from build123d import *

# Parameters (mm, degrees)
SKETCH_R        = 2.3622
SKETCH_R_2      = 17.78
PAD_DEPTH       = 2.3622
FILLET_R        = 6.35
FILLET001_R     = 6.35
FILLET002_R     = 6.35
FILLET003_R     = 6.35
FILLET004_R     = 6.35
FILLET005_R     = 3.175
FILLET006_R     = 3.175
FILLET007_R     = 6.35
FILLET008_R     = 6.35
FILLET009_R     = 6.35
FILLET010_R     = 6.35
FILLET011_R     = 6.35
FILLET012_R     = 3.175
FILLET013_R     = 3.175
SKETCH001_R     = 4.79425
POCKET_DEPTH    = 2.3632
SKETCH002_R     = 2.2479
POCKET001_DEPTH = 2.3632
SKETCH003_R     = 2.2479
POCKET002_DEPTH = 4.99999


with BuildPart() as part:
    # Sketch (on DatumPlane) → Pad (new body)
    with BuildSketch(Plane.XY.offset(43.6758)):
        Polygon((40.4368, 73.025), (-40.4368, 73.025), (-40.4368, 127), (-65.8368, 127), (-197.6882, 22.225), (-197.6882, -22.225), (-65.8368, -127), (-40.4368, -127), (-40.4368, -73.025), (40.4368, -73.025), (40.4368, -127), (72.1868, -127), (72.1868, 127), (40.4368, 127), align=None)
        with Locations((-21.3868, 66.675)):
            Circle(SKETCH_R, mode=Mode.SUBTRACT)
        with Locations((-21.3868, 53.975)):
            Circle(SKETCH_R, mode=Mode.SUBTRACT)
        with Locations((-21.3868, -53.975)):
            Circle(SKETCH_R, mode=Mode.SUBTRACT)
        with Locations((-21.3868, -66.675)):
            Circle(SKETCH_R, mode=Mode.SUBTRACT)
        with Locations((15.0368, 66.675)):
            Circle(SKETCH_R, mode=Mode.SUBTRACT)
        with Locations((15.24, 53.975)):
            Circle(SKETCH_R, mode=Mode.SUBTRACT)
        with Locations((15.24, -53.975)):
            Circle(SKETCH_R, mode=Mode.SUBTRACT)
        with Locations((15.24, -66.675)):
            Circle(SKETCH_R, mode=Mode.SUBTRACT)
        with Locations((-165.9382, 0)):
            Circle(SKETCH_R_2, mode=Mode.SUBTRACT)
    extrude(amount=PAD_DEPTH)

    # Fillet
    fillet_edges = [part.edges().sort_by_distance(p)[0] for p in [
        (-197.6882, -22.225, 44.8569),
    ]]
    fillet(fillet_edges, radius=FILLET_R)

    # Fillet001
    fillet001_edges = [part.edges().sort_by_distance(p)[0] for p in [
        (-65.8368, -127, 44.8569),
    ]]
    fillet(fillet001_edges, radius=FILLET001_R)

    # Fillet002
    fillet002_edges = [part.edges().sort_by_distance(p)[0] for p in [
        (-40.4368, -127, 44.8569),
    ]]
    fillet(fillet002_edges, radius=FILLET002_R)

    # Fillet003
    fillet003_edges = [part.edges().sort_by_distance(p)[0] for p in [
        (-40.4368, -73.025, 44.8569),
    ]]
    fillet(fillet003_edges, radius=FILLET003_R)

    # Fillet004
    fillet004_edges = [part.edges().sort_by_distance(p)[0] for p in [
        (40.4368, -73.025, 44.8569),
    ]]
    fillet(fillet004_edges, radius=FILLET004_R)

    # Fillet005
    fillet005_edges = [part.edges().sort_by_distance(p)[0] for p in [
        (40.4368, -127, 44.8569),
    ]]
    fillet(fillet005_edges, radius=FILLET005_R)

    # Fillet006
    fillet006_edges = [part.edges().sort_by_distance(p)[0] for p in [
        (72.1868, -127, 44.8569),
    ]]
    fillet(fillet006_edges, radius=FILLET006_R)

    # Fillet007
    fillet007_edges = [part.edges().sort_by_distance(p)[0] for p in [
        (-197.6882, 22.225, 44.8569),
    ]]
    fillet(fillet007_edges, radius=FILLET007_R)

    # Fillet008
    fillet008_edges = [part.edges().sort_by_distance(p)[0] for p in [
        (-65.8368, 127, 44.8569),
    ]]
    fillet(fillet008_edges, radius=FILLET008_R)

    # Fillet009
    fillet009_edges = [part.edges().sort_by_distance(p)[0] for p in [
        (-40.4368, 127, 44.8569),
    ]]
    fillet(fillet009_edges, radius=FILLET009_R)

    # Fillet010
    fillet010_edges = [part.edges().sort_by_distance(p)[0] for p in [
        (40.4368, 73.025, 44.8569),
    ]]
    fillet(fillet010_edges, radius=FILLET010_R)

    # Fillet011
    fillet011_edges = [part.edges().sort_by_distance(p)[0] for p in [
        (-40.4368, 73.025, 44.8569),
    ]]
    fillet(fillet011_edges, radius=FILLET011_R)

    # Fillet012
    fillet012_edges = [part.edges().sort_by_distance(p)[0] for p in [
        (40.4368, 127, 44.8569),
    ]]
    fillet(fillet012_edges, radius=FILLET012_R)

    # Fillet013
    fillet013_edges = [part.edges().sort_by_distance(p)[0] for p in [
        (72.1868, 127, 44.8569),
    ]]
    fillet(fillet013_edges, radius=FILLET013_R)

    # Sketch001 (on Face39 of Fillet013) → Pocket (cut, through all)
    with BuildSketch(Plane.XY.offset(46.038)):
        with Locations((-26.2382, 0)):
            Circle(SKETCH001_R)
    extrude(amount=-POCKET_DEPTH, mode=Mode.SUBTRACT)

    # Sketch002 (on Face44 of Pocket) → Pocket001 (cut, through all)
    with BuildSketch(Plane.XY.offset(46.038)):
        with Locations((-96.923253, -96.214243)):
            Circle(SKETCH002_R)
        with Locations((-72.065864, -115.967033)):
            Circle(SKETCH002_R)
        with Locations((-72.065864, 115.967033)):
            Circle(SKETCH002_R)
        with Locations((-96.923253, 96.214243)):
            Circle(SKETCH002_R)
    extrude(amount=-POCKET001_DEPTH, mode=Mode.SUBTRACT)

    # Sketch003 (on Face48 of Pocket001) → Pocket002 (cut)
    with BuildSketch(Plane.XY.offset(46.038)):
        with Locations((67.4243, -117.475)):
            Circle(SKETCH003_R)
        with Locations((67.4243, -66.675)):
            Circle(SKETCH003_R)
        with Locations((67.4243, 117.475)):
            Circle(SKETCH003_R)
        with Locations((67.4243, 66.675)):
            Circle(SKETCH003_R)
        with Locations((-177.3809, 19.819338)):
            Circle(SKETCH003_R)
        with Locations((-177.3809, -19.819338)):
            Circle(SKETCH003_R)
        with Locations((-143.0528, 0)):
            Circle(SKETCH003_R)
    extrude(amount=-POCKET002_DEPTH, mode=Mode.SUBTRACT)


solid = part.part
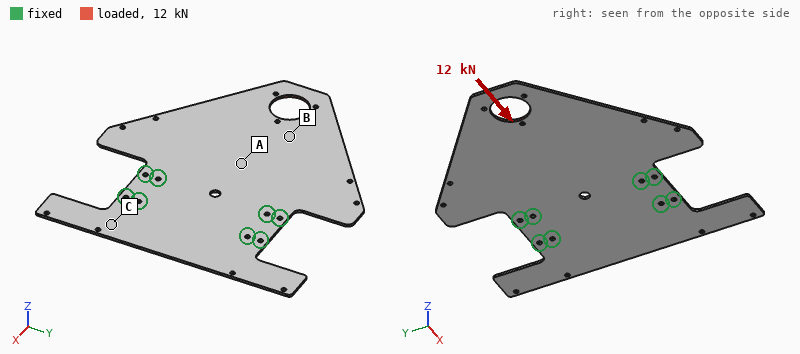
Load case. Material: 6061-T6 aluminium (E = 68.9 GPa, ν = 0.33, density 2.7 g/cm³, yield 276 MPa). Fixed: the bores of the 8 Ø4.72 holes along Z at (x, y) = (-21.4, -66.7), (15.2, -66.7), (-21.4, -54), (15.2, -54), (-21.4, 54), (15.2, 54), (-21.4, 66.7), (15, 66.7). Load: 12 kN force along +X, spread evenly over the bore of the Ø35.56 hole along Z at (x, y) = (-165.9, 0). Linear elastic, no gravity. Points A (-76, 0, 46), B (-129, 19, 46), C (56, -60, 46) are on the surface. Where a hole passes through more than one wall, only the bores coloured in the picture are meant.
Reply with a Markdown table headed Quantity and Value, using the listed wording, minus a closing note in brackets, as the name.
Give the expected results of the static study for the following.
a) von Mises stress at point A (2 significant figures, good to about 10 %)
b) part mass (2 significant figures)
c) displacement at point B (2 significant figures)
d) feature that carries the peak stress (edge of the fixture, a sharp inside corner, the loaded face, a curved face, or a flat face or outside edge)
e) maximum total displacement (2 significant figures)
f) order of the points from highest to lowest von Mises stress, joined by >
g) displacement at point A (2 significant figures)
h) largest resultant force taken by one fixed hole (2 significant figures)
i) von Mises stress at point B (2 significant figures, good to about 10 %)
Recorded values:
| Quantity | Value |
|---|---|
| von Mises stress at point A | 33 MPa |
| part mass | 280 g |
| displacement at point B | 0.071 mm |
| feature that carries the peak stress | a curved face |
| maximum total displacement | 0.16 mm |
| order of the points from highest to lowest von Mises stress, joined by > | B > A > C |
| displacement at point A | 0.040 mm |
| largest resultant force taken by one fixed hole | 2.6 kN |
| von Mises stress at point B | 52 MPa |
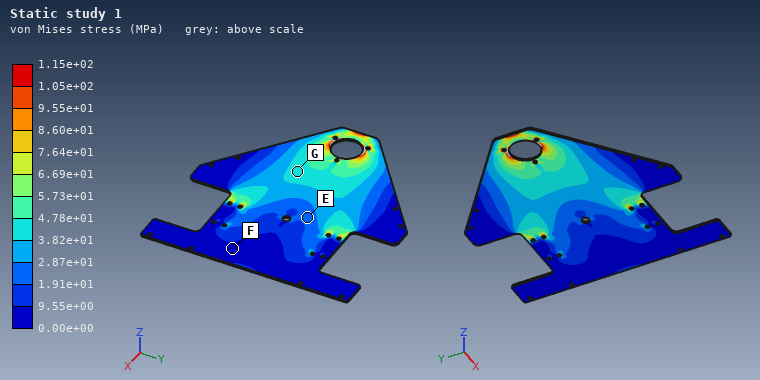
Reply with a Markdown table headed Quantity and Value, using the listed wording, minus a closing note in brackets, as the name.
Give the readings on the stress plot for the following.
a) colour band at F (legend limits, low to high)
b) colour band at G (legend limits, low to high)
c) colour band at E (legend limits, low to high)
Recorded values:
| Quantity | Value |
|---|---|
| colour band at F | 0.00e+00 to 9.55e+00 MPa |
| colour band at G | 3.82e+01 to 4.78e+01 MPa |
| colour band at E | 1.91e+01 to 2.87e+01 MPa |
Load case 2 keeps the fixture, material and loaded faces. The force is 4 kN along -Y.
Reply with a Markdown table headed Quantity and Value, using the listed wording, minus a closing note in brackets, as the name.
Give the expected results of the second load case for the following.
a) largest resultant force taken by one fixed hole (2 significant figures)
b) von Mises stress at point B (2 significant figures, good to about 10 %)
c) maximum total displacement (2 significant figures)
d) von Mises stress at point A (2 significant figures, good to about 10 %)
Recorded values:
| Quantity | Value |
|---|---|
| largest resultant force taken by one fixed hole | 2.6 kN |
| von Mises stress at point B | 22 MPa |
| maximum total displacement | 0.21 mm |
| von Mises stress at point A | 29 MPa |
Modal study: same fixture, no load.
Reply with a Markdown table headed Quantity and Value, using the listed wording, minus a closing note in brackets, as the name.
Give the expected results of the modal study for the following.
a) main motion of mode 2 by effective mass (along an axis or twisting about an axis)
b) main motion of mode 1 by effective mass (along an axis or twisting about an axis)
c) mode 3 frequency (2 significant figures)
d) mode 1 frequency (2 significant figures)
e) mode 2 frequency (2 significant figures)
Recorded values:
| Quantity | Value |
|---|---|
| main motion of mode 2 by effective mass | twisting about X |
| main motion of mode 1 by effective mass | along Z |
| mode 3 frequency | 300 Hz |
| mode 1 frequency | 83 Hz |
| mode 2 frequency | 200 Hz |
